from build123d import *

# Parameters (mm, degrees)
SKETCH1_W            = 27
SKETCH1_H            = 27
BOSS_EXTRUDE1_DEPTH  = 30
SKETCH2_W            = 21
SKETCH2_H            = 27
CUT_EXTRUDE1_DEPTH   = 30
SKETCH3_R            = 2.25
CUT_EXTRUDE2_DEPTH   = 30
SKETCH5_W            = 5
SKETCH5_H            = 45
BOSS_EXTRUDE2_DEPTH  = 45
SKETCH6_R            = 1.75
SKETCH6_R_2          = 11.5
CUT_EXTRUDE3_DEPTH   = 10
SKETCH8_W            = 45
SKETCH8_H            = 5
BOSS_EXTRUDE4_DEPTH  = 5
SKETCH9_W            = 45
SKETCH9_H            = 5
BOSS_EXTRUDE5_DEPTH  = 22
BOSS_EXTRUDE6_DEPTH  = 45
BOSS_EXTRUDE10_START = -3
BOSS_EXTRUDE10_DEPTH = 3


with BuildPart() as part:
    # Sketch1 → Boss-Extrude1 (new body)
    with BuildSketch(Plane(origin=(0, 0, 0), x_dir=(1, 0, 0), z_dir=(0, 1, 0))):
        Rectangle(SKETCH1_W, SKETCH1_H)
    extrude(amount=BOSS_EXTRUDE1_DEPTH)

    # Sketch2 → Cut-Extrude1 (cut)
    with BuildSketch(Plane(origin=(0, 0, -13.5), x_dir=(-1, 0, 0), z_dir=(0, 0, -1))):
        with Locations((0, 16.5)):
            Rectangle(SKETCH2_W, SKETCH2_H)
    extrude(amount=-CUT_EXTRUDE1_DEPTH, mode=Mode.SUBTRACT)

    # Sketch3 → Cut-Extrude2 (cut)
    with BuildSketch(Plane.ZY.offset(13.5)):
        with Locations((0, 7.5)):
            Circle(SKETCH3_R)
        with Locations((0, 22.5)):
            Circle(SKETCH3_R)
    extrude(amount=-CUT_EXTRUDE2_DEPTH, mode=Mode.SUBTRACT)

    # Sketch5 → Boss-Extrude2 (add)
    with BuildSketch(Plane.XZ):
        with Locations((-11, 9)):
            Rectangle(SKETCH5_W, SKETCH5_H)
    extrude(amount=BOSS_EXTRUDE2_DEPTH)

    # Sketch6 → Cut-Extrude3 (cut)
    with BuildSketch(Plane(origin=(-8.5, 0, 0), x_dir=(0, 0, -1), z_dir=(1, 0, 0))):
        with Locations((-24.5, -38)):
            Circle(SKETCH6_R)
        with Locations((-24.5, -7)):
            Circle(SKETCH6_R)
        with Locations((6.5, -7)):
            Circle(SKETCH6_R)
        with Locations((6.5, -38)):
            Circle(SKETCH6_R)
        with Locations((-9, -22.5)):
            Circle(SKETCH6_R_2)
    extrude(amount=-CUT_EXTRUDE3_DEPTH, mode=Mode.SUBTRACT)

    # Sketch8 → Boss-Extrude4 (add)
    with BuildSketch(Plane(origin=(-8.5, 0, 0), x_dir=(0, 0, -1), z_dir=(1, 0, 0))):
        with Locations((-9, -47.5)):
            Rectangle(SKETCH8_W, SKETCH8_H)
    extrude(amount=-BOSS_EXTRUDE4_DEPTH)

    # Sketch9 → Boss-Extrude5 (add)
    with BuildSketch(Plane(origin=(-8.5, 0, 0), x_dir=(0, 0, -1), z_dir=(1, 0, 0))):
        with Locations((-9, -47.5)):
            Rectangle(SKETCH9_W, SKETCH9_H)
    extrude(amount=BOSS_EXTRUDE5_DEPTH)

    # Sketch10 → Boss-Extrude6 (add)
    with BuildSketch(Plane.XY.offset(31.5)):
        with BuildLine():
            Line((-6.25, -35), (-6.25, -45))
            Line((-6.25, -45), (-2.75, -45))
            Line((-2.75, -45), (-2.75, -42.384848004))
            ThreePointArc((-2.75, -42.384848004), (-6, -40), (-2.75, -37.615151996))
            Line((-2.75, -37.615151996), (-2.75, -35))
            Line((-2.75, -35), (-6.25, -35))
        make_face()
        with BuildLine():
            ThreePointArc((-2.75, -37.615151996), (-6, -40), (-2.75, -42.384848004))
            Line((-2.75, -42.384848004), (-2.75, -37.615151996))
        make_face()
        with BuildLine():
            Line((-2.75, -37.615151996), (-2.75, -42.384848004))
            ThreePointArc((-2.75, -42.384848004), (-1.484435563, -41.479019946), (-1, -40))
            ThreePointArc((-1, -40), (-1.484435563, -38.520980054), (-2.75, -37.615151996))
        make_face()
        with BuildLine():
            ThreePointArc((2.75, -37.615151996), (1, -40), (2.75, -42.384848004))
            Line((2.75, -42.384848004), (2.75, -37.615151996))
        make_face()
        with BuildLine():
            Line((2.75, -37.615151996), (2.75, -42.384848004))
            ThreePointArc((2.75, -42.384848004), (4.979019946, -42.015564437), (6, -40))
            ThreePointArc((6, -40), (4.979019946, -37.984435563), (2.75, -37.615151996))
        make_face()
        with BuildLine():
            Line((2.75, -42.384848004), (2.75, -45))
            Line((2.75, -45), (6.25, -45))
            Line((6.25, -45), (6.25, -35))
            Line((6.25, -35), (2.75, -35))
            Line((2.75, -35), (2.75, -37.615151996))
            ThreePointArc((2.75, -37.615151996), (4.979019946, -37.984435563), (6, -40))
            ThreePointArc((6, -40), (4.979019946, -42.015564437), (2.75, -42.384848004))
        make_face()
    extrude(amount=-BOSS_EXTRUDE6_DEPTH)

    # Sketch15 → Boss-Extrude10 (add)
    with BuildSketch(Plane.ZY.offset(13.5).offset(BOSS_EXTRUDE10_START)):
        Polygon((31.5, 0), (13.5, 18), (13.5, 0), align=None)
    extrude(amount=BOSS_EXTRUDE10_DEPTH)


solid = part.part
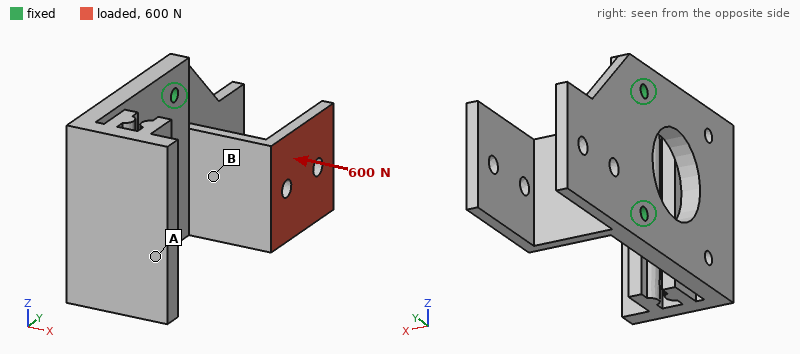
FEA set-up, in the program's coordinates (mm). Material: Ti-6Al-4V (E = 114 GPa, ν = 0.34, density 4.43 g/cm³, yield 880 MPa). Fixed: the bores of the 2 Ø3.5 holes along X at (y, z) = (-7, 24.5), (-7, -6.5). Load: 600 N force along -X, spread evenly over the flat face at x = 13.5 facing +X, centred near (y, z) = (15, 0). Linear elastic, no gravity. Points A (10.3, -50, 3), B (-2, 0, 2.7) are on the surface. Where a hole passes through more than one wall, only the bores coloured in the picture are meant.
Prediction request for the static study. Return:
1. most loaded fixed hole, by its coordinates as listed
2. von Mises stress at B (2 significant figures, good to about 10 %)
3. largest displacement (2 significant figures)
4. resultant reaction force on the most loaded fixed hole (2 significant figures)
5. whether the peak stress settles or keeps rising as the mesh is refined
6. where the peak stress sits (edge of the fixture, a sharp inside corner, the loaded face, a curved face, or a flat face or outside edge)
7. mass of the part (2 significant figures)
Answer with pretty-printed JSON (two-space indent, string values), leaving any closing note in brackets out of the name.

{
  "most loaded fixed hole, by its coordinates as listed": "(-7, -6.5)",
  "von Mises stress at B": "170 MPa",
  "largest displacement": "1.1 mm",
  "resultant reaction force on the most loaded fixed hole": "450 N",
  "whether the peak stress settles or keeps rising as the mesh is refined": "keeps rising",
  "where the peak stress sits": "edge of the fixture",
  "mass of the part": "110 g"
}
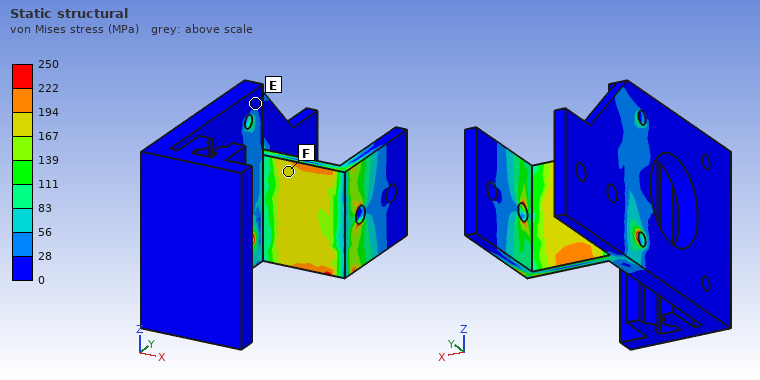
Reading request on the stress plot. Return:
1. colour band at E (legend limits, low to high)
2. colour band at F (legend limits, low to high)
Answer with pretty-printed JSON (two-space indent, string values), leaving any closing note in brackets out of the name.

{
  "colour band at E": "0 to 28 MPa",
  "colour band at F": "167 to 194 MPa"
}
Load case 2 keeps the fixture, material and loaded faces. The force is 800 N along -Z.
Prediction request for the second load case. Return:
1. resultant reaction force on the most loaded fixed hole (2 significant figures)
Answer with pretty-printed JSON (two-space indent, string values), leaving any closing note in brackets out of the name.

{
  "resultant reaction force on the most loaded fixed hole": "940 N"
}
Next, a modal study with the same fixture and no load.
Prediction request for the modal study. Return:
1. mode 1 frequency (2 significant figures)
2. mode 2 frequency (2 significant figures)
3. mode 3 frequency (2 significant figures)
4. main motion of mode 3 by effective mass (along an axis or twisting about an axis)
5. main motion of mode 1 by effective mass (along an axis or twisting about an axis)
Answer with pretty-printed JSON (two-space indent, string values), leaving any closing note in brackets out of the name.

{
  "mode 1 frequency": "830 Hz",
  "mode 2 frequency": "1200 Hz",
  "mode 3 frequency": "1800 Hz",
  "main motion of mode 3 by effective mass": "along Z",
  "main motion of mode 1 by effective mass": "along X"
}
